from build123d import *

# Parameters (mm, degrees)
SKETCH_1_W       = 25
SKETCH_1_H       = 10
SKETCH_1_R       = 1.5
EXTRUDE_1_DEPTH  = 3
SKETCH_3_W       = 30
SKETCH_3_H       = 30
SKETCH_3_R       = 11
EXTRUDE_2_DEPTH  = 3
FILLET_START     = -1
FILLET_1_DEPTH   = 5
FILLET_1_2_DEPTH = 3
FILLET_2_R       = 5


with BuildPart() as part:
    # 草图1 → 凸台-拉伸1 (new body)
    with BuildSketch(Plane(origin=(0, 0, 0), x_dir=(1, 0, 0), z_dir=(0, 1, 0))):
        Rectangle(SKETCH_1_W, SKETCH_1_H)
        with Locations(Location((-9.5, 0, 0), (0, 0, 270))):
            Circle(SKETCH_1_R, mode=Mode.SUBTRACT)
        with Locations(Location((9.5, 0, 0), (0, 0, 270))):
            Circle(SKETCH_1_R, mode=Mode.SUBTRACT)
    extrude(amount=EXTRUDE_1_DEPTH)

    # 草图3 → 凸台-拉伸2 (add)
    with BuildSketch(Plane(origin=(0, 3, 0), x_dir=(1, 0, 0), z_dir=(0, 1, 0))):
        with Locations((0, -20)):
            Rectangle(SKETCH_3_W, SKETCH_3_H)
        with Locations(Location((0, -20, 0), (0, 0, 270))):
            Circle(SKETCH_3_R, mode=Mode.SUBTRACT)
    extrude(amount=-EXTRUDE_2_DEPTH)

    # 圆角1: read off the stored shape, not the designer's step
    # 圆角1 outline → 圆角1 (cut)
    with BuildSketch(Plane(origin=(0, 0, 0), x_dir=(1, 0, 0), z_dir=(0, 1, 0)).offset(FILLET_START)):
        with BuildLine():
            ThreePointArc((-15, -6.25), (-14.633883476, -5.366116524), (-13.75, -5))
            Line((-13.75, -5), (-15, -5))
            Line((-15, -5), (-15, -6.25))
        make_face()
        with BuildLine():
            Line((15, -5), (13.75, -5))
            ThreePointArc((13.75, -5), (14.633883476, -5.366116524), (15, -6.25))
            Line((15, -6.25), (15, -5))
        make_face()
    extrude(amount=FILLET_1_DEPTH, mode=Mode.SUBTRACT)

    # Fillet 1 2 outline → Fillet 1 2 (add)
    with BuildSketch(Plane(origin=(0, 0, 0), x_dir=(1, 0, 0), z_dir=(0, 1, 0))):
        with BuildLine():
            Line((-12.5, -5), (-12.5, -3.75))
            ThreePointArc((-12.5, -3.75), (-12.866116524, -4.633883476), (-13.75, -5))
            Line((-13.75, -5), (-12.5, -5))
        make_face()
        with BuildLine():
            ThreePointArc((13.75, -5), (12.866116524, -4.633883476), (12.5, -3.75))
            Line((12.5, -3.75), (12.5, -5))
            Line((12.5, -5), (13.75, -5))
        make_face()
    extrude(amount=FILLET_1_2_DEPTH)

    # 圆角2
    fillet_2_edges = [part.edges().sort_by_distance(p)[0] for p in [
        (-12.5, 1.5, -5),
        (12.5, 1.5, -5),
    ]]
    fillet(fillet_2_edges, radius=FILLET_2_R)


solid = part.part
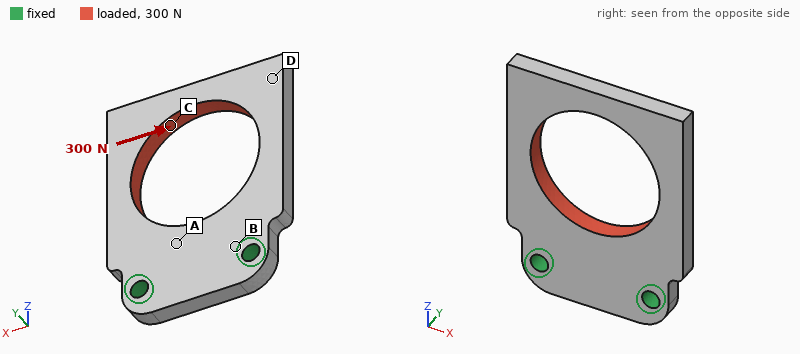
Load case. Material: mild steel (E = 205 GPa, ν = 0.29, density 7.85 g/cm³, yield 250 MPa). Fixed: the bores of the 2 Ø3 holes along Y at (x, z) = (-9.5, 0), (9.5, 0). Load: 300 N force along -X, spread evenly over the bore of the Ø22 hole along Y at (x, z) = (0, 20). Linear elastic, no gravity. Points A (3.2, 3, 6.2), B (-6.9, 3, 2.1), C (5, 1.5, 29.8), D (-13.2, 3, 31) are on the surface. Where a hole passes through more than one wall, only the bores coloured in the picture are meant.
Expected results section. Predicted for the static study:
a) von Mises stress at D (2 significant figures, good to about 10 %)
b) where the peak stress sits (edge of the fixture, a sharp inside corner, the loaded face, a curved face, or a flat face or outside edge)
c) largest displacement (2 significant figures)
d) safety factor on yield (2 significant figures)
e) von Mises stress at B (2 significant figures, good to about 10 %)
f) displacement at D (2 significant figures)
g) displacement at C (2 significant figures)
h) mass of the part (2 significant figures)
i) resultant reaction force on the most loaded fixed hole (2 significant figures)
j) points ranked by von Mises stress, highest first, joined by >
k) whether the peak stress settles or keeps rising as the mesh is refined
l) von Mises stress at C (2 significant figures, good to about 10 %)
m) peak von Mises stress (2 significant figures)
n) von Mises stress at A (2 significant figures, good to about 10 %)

8.2 MPa
a curved face
14 µm
4.1
12 MPa
13 µm
13 µm
18 g
330 N
C > A > B > D
settles
26 MPa
62 MPa
19 MPa
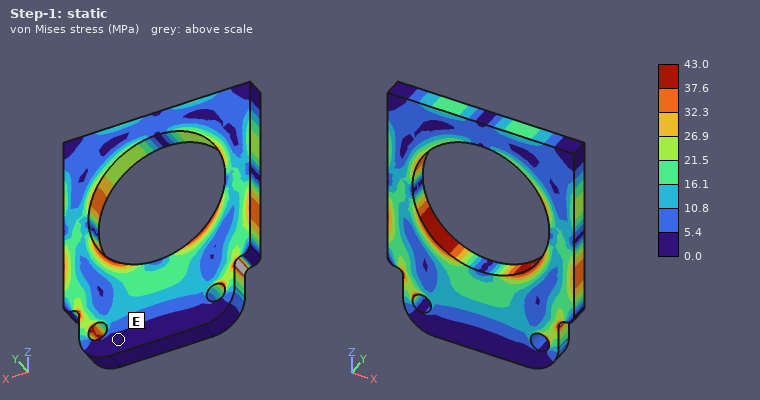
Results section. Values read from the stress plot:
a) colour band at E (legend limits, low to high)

0.0 to 5.4 MPa
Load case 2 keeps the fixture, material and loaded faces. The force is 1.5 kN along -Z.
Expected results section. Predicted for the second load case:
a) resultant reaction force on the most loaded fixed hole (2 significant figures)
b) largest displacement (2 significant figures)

760 N
14 µm
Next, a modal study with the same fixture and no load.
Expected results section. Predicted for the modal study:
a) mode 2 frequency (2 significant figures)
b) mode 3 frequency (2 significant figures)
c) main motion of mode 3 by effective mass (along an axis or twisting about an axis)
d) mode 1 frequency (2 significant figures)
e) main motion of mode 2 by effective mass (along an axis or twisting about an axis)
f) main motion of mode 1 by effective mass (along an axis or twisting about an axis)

4100 Hz
7300 Hz
along X
1800 Hz
twisting about Z
along Y
